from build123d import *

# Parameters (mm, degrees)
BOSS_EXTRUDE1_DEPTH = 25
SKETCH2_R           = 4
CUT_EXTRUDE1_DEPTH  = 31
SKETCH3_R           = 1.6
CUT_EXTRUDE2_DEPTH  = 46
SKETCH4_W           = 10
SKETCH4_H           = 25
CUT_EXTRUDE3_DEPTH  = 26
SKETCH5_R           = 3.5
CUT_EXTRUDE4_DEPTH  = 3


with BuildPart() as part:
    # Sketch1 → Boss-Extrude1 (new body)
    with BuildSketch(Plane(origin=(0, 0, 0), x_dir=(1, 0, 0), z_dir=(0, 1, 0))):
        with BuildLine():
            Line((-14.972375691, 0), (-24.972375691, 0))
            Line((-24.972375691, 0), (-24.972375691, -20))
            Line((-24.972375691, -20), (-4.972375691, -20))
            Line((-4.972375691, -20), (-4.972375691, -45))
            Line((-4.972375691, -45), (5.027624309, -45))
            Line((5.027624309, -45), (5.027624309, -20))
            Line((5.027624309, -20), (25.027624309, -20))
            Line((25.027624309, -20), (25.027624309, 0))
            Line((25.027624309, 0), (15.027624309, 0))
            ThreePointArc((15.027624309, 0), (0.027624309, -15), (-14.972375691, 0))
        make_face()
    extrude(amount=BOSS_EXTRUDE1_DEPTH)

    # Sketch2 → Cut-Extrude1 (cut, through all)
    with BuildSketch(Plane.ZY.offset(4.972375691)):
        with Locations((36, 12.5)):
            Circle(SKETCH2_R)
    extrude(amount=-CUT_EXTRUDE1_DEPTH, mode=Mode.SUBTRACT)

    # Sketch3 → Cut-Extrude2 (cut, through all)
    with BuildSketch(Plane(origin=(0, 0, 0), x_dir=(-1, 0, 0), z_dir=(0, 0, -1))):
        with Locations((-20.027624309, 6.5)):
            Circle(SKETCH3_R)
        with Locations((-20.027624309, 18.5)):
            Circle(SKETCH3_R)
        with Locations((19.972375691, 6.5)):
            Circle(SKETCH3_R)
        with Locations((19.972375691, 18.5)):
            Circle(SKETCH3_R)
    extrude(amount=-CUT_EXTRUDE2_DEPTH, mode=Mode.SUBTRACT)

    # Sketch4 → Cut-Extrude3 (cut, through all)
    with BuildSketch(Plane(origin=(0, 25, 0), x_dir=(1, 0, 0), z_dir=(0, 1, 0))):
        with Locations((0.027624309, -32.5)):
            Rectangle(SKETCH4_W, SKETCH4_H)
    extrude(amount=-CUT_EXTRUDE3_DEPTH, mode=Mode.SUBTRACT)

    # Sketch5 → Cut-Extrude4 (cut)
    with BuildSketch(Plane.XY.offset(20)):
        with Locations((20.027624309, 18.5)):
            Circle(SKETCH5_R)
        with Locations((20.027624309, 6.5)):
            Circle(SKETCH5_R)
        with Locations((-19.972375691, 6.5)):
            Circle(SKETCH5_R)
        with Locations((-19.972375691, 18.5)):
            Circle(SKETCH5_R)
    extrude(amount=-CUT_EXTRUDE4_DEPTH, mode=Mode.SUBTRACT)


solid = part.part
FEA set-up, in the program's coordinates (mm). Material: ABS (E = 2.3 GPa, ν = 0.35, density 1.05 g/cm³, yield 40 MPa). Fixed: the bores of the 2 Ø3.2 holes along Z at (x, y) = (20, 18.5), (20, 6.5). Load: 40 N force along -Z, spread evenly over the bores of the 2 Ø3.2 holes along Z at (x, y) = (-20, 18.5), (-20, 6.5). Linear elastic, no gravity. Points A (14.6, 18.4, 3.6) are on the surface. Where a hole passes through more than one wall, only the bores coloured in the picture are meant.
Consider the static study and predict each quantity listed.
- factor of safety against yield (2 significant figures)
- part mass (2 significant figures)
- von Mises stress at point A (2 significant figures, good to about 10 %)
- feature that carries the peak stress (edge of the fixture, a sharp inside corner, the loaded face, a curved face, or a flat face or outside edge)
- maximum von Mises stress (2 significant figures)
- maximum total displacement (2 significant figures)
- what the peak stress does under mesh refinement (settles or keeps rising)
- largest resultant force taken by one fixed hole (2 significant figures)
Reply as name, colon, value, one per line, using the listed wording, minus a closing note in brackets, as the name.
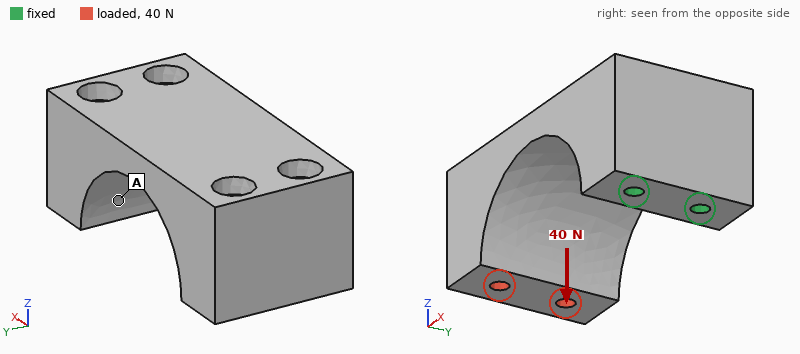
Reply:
factor of safety against yield: 5.1
part mass: 16 g
von Mises stress at point A: 0.87 MPa
feature that carries the peak stress: a flat face or outside edge
maximum von Mises stress: 7.8 MPa
maximum total displacement: 0.65 mm
what the peak stress does under mesh refinement: settles
largest resultant force taken by one fixed hole: 21 N
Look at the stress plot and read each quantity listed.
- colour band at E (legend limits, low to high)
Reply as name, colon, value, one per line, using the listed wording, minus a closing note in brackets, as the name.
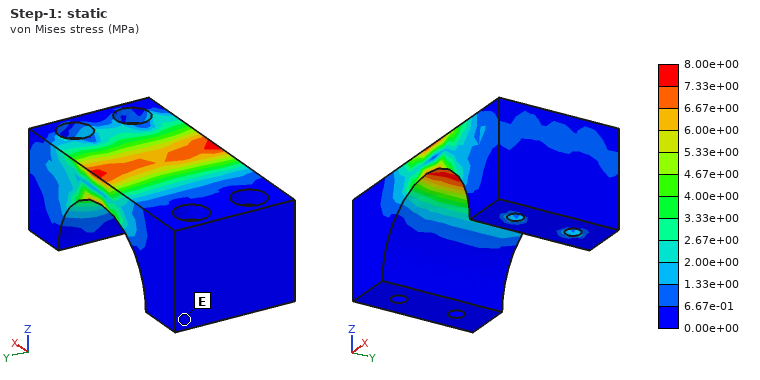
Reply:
colour band at E: 0.00e+00 to 6.67e-01 MPa
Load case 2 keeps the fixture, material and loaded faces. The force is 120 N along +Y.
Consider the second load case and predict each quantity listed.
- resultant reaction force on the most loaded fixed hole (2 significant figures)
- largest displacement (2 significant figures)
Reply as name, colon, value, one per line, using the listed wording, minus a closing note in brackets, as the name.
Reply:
resultant reaction force on the most loaded fixed hole: 330 N
largest displacement: 0.51 mm
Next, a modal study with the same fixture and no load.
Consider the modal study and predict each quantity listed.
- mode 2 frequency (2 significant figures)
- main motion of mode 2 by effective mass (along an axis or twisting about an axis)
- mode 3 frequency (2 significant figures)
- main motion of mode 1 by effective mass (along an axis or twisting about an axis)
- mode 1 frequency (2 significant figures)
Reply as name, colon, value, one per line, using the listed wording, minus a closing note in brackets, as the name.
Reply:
mode 2 frequency: 1200 Hz
main motion of mode 2 by effective mass: along Y
mode 3 frequency: 2400 Hz
main motion of mode 1 by effective mass: along Z
mode 1 frequency: 580 Hz
